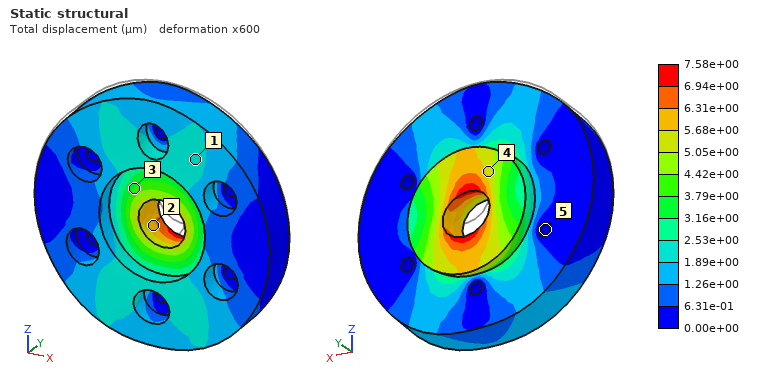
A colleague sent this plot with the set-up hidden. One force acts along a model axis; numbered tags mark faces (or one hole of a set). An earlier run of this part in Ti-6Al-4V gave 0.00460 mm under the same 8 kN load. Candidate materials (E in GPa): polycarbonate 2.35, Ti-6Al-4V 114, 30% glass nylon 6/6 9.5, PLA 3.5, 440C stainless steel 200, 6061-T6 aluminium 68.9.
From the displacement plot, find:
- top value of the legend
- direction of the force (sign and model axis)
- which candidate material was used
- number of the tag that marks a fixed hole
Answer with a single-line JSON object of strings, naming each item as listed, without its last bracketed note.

{"top value of the legend": "7.58e+00 µm", "direction of the force": "-Z", "which candidate material was used": "6061-T6 aluminium", "number of the tag that marks a fixed hole": "5"}
